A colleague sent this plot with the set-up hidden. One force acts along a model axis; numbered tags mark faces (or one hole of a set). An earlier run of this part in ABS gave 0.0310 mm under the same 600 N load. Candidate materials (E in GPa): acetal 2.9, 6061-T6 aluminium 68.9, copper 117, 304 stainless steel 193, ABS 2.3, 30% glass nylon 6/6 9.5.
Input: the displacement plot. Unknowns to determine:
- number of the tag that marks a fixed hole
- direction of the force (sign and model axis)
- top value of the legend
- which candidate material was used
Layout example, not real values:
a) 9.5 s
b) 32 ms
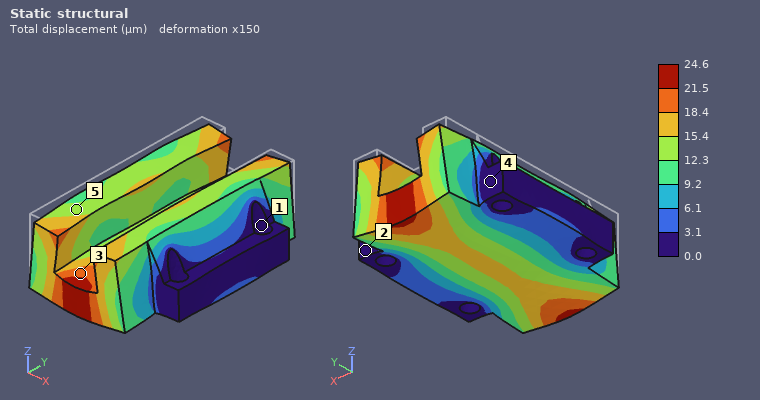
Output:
a) 1
b) -Z
c) 24.6 µm
d) acetal
